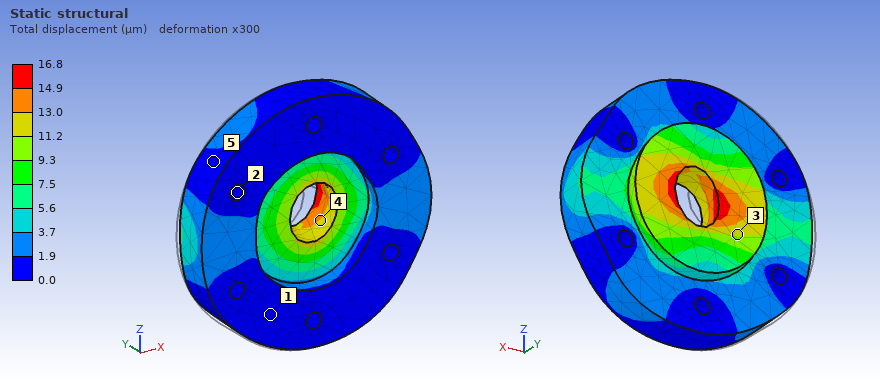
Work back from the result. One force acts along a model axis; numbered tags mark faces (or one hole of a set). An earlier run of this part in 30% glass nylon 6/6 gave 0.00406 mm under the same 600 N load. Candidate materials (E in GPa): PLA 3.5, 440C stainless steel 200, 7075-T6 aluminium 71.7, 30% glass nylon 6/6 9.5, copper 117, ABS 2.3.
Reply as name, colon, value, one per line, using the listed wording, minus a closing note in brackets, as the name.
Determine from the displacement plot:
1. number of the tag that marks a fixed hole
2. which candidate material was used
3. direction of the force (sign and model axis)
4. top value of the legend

number of the tag that marks a fixed hole: 2
which candidate material was used: ABS
direction of the force: +X
top value of the legend: 16.8 µm
